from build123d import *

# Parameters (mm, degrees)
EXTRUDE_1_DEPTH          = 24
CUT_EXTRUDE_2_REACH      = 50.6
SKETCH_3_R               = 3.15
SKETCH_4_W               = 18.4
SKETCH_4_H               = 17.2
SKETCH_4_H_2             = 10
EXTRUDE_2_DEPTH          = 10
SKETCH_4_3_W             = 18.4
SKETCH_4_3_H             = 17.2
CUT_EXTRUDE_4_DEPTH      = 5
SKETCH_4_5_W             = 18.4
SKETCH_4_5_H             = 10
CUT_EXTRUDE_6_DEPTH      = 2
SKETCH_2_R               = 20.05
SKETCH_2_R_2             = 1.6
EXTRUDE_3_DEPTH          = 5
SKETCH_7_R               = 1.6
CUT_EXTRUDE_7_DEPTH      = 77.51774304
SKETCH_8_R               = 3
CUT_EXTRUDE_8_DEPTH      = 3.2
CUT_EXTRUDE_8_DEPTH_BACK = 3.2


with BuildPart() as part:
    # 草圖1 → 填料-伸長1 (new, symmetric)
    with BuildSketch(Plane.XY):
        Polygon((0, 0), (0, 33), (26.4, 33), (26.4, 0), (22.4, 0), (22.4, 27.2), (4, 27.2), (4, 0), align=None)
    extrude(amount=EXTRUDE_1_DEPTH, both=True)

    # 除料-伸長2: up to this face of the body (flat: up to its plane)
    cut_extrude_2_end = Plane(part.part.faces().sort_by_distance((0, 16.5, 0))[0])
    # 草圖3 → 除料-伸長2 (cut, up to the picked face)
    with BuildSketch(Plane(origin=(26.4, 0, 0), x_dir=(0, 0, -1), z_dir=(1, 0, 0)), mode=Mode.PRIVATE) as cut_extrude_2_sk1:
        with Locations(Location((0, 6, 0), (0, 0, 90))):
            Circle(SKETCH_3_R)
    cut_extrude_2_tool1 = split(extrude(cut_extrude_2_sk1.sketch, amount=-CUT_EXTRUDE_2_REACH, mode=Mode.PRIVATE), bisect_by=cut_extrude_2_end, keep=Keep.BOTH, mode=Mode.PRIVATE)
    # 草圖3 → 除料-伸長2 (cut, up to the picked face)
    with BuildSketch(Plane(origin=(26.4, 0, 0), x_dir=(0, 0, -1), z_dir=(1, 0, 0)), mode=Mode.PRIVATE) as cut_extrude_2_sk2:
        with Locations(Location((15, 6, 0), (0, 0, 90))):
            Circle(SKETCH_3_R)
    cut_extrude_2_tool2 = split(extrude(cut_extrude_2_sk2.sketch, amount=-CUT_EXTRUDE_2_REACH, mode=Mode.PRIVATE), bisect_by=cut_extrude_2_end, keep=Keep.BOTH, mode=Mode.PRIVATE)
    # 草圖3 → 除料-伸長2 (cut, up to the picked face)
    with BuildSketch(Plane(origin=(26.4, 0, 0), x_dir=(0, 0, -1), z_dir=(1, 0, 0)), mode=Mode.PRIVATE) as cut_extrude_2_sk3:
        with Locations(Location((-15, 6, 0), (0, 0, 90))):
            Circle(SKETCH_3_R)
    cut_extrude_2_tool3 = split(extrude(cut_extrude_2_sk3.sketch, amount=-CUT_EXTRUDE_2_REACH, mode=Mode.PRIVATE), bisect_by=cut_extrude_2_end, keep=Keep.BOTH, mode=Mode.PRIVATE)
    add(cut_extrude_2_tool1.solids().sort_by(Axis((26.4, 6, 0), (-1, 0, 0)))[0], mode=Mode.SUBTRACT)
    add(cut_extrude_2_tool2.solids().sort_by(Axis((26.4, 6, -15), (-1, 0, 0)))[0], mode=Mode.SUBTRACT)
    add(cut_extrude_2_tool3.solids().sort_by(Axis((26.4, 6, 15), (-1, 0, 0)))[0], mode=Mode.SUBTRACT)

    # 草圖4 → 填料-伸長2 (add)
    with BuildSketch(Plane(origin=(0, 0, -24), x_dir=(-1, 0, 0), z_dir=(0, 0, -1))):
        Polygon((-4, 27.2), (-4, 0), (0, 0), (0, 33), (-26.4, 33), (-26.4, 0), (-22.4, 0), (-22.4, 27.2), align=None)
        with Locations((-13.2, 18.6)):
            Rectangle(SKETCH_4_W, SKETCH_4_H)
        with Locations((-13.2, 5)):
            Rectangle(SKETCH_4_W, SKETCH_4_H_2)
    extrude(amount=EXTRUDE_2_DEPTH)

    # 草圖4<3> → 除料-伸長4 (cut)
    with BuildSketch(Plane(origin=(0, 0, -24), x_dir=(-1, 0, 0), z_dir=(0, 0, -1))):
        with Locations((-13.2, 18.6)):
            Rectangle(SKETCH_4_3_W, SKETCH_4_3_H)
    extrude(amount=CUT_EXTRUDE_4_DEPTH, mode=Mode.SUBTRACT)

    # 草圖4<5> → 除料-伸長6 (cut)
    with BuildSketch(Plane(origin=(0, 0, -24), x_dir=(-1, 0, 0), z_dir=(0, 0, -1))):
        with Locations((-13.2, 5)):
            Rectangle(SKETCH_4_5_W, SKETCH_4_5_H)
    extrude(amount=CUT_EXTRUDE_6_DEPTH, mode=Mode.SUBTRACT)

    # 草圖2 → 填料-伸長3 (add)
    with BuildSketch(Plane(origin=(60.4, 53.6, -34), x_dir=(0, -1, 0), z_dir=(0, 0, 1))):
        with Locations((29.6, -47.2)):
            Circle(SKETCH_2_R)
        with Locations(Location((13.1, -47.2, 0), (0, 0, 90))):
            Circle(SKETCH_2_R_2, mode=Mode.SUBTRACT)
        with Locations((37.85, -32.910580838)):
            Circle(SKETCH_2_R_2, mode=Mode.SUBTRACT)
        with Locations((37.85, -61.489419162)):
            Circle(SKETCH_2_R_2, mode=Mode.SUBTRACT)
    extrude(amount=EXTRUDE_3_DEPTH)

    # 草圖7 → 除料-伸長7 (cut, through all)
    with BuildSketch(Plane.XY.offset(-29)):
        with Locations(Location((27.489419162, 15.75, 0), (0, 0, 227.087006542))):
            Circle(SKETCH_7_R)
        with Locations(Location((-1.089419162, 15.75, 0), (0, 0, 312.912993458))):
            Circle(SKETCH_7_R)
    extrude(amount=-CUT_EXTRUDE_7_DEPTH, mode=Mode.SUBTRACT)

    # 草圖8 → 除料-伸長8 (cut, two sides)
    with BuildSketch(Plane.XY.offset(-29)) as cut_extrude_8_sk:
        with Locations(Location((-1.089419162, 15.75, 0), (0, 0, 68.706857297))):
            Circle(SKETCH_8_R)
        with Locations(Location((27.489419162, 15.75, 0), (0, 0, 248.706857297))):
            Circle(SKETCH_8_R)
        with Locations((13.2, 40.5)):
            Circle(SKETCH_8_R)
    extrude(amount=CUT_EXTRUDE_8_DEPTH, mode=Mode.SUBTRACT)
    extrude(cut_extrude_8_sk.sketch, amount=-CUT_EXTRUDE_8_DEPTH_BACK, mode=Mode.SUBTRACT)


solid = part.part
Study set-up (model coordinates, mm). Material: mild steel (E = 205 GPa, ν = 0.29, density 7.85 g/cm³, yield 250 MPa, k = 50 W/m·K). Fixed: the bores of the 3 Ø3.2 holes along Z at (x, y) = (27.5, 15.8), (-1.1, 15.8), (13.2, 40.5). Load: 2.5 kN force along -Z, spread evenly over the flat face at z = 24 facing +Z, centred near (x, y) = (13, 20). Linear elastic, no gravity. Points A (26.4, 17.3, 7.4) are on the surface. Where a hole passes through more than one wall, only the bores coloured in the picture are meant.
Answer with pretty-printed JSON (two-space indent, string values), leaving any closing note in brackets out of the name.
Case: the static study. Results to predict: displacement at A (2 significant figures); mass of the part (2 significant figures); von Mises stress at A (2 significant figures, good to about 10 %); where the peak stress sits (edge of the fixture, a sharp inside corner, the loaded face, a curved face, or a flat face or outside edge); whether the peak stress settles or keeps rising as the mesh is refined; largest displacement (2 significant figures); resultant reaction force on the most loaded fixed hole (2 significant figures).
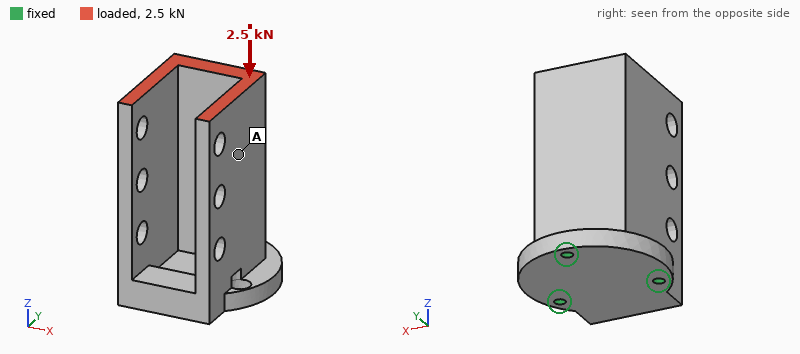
{
  "displacement at A": "4.5 µm",
  "mass of the part": "210 g",
  "von Mises stress at A": "8.4 MPa",
  "where the peak stress sits": "edge of the fixture",
  "whether the peak stress settles or keeps rising as the mesh is refined": "keeps rising",
  "largest displacement": "5.8 µm",
  "resultant reaction force on the most loaded fixed hole": "1.1 kN"
}
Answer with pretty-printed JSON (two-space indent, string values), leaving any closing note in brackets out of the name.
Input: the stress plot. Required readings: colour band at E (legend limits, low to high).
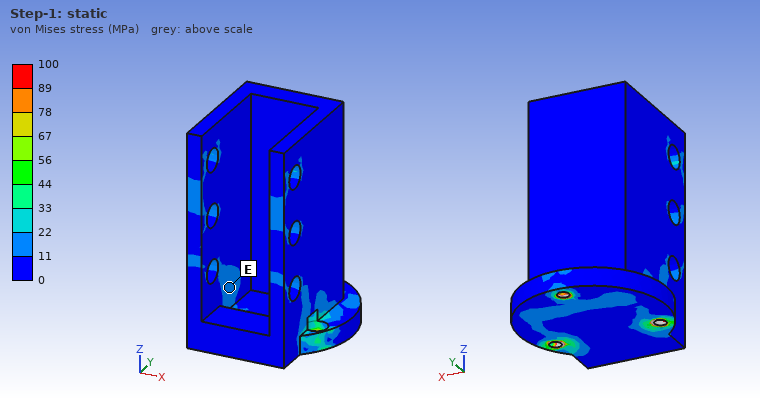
{
  "colour band at E": "11 to 22 MPa"
}
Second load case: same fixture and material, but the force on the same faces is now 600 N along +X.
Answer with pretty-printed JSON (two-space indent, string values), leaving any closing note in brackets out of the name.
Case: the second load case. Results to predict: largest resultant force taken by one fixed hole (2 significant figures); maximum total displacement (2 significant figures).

{
  "largest resultant force taken by one fixed hole": "1.3 kN",
  "maximum total displacement": "93 µm"
}
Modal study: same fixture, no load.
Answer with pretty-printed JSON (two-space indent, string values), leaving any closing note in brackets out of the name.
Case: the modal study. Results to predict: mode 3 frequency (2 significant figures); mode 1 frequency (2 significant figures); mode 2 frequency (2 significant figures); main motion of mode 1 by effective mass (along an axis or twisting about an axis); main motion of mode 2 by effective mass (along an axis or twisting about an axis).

{
  "mode 3 frequency": "4600 Hz",
  "mode 1 frequency": "2300 Hz",
  "mode 2 frequency": "2700 Hz",
  "main motion of mode 1 by effective mass": "along X",
  "main motion of mode 2 by effective mass": "along Y"
}
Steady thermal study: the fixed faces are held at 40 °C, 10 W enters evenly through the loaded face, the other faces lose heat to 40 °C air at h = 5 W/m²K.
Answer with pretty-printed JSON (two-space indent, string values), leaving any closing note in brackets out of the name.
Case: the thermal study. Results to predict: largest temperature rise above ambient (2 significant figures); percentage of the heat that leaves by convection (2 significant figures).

{
  "largest temperature rise above ambient": "39 K",
  "percentage of the heat that leaves by convection": "12 %"
}
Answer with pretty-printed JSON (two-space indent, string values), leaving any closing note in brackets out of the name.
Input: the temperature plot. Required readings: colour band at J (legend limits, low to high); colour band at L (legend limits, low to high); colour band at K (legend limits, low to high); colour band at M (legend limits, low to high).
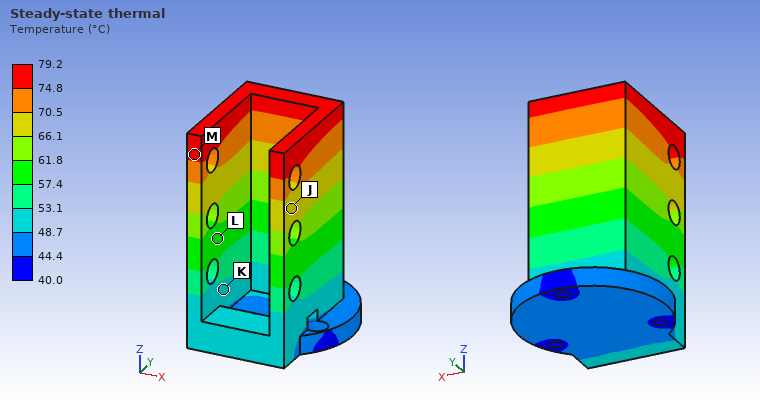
{
  "colour band at J": "66.1 to 70.5 °C",
  "colour band at L": "57.4 to 61.8 °C",
  "colour band at K": "48.7 to 53.1 °C",
  "colour band at M": "74.8 to 79.2 °C"
}
